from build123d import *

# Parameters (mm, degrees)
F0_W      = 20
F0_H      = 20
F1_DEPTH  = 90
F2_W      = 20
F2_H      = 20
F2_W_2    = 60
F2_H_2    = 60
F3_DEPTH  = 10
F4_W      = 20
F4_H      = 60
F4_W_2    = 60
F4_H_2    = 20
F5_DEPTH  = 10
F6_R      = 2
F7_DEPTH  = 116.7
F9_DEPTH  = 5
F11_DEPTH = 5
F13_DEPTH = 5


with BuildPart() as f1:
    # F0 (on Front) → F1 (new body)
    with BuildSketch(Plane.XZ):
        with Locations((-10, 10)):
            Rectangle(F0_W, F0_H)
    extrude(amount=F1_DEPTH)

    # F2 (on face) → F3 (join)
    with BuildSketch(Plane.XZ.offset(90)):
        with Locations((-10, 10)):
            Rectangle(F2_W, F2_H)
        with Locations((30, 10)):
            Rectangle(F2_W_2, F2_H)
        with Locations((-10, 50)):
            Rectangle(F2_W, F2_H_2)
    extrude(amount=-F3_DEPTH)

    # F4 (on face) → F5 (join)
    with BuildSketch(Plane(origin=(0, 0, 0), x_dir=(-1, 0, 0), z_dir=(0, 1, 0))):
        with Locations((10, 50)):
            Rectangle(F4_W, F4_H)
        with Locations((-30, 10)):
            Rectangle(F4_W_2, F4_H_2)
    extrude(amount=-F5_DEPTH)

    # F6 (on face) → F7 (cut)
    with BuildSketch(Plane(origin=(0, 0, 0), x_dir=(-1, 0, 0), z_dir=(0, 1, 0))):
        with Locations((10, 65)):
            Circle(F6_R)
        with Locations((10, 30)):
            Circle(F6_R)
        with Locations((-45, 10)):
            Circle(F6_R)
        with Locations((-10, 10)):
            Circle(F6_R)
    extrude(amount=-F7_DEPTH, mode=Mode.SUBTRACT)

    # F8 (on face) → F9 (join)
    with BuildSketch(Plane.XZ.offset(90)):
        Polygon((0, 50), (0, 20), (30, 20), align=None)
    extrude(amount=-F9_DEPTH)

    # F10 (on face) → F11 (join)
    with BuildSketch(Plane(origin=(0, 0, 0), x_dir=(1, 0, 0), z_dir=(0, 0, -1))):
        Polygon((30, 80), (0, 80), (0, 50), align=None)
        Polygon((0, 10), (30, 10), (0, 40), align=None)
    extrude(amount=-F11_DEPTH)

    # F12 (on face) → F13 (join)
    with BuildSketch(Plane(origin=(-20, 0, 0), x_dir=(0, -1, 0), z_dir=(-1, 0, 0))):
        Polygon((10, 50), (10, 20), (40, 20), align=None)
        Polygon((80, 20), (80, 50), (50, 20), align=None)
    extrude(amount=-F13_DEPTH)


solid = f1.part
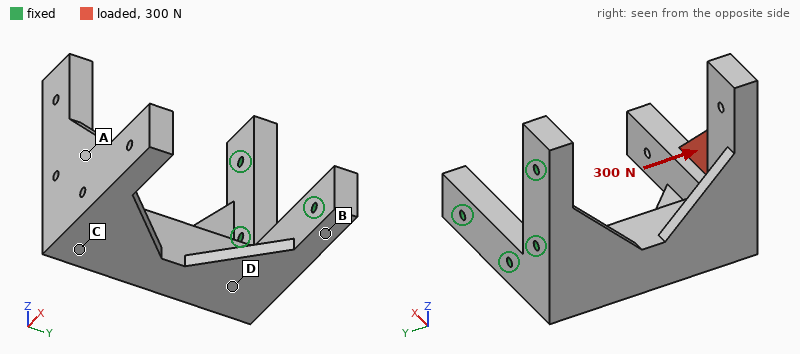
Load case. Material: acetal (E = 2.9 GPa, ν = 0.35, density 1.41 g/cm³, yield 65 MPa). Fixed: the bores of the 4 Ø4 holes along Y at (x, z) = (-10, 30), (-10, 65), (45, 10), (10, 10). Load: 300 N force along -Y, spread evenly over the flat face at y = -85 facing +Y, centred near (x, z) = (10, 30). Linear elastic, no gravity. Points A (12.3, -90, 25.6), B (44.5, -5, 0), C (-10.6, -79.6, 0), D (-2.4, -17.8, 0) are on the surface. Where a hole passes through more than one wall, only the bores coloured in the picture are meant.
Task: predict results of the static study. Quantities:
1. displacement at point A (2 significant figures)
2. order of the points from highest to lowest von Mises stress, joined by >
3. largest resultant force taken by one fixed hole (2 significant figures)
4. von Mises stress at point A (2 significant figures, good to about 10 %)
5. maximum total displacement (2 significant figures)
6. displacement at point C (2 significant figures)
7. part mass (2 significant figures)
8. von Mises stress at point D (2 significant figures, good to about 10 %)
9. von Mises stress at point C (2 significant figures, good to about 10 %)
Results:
1.1 mm
A > C > D > B
100 N
4.1 MPa
1.5 mm
0.76 mm
130 g
1.8 MPa
3.0 MPa
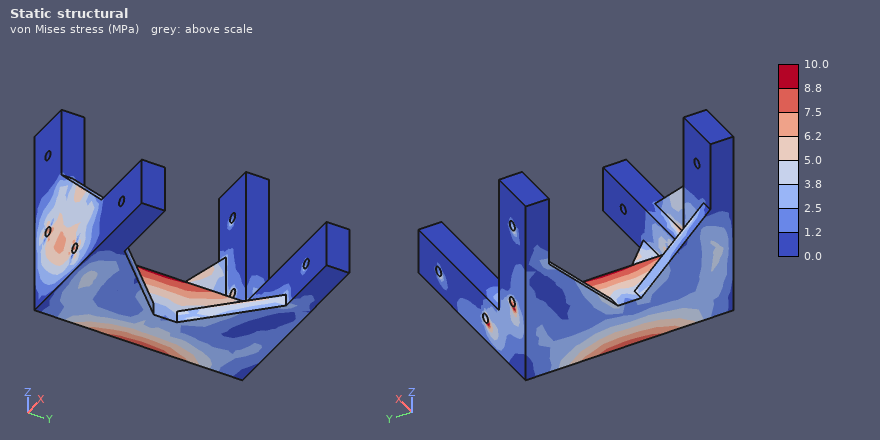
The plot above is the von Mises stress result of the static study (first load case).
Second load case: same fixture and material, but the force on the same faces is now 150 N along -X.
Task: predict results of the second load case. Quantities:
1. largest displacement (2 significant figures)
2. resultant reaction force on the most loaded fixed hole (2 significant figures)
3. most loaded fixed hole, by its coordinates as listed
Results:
1.7 mm
300 N
(-10, 30)
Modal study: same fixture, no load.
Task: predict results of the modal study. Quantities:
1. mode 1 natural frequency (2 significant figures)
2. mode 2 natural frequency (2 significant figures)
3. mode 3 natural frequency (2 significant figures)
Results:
220 Hz
280 Hz
510 Hz
